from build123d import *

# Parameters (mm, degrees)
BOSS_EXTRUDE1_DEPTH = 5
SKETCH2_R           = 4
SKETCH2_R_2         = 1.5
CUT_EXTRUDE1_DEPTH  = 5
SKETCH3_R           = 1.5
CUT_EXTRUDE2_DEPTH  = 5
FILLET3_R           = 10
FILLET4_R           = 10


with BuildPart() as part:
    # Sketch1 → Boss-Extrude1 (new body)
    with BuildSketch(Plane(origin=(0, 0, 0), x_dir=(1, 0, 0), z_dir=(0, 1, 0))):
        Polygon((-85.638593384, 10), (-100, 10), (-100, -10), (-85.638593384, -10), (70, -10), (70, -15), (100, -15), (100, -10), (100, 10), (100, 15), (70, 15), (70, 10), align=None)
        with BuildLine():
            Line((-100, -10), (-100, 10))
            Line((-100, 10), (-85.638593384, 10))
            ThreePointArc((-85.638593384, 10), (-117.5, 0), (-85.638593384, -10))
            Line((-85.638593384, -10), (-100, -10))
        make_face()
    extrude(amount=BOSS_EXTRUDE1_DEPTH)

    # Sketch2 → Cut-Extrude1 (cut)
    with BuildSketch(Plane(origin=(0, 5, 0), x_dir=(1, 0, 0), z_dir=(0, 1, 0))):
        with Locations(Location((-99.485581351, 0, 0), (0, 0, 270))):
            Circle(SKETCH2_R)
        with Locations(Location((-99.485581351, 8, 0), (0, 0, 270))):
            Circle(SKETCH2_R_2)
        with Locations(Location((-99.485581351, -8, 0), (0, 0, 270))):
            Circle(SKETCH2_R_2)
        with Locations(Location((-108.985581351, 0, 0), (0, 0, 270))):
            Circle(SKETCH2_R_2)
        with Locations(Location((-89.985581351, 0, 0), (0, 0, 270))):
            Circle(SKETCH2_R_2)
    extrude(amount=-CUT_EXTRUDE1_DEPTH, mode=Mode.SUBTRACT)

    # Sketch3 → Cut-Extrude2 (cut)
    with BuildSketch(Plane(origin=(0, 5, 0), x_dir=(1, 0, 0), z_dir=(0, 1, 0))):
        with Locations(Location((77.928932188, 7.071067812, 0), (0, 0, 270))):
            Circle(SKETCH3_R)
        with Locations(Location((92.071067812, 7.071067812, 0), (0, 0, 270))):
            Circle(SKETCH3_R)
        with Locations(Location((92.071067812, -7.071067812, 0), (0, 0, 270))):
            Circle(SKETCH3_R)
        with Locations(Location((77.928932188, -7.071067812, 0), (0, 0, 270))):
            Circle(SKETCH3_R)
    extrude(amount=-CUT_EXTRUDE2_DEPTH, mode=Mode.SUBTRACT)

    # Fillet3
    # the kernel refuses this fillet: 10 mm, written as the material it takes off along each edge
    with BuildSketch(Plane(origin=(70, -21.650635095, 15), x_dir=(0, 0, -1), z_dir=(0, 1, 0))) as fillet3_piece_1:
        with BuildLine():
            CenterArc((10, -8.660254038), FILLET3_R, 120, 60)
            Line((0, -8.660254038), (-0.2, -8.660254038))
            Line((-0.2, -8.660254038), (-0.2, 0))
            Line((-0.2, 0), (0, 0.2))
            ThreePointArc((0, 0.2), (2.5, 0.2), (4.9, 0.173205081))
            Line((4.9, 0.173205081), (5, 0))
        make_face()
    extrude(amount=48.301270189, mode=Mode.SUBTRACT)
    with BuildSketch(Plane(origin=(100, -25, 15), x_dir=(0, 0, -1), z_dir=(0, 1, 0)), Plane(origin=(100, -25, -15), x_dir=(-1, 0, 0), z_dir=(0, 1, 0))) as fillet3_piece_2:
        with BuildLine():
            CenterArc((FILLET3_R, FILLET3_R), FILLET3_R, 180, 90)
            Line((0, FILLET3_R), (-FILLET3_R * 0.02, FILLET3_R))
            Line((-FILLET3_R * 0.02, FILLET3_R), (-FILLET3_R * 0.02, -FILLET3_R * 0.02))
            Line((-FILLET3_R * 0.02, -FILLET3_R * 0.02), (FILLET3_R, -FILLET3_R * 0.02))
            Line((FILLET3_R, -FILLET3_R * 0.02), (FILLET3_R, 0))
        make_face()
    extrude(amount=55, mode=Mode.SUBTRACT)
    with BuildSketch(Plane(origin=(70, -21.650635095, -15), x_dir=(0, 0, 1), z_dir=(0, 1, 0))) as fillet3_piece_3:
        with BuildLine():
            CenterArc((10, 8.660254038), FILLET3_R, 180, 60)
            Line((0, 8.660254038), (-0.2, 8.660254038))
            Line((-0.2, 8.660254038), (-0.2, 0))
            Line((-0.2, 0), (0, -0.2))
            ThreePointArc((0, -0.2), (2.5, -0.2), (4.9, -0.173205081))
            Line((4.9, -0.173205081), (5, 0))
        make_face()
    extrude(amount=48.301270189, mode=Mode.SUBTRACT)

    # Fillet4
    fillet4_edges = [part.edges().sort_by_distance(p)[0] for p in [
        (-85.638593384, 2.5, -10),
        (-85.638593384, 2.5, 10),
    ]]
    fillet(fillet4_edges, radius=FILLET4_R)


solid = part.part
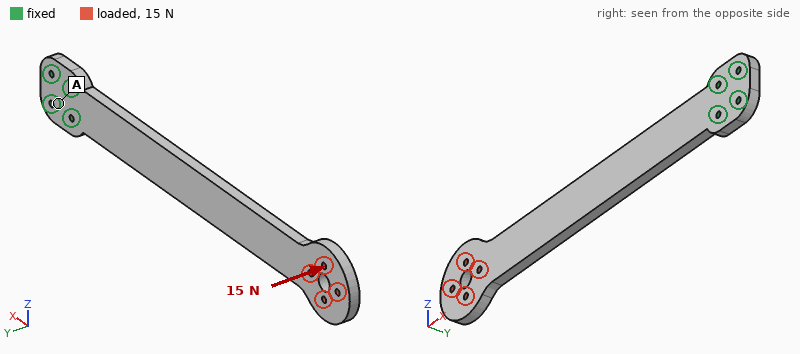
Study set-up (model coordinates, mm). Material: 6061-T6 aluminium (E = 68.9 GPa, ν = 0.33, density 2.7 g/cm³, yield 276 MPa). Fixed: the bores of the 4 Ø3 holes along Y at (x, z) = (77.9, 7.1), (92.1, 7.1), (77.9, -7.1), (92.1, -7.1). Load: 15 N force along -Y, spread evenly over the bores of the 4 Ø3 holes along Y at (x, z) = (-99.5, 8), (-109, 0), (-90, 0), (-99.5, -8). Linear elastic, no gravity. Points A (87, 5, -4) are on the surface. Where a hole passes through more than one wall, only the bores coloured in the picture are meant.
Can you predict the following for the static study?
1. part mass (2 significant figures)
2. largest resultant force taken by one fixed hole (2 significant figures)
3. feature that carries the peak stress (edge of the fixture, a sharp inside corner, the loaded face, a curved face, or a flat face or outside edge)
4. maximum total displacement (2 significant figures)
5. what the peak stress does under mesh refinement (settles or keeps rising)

64 g
35 N
edge of the fixture
2.2 mm
keeps rising
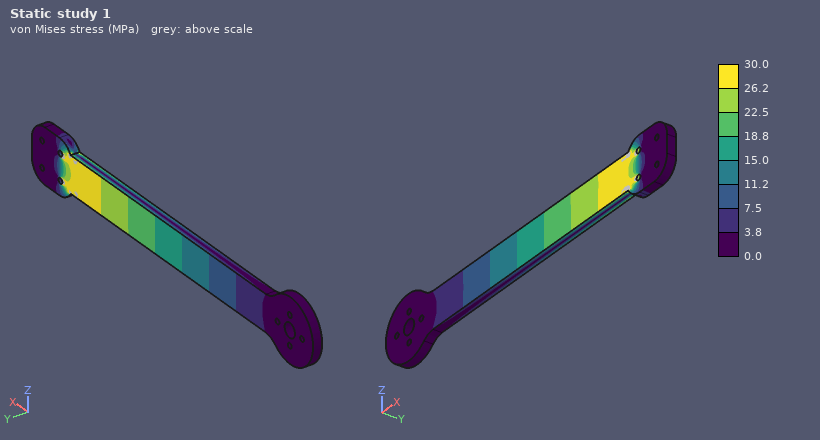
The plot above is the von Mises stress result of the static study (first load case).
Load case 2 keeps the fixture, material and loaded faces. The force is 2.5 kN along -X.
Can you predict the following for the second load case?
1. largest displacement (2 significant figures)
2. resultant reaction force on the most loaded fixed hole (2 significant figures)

66 µm
1.1 kN
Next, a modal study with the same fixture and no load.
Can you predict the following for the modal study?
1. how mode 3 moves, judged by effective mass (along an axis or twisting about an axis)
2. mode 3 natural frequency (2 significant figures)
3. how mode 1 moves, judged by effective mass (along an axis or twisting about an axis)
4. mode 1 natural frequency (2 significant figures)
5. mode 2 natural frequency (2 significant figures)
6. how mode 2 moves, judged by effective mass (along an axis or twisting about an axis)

along Y
660 Hz
along Y
100 Hz
400 Hz
along Z
